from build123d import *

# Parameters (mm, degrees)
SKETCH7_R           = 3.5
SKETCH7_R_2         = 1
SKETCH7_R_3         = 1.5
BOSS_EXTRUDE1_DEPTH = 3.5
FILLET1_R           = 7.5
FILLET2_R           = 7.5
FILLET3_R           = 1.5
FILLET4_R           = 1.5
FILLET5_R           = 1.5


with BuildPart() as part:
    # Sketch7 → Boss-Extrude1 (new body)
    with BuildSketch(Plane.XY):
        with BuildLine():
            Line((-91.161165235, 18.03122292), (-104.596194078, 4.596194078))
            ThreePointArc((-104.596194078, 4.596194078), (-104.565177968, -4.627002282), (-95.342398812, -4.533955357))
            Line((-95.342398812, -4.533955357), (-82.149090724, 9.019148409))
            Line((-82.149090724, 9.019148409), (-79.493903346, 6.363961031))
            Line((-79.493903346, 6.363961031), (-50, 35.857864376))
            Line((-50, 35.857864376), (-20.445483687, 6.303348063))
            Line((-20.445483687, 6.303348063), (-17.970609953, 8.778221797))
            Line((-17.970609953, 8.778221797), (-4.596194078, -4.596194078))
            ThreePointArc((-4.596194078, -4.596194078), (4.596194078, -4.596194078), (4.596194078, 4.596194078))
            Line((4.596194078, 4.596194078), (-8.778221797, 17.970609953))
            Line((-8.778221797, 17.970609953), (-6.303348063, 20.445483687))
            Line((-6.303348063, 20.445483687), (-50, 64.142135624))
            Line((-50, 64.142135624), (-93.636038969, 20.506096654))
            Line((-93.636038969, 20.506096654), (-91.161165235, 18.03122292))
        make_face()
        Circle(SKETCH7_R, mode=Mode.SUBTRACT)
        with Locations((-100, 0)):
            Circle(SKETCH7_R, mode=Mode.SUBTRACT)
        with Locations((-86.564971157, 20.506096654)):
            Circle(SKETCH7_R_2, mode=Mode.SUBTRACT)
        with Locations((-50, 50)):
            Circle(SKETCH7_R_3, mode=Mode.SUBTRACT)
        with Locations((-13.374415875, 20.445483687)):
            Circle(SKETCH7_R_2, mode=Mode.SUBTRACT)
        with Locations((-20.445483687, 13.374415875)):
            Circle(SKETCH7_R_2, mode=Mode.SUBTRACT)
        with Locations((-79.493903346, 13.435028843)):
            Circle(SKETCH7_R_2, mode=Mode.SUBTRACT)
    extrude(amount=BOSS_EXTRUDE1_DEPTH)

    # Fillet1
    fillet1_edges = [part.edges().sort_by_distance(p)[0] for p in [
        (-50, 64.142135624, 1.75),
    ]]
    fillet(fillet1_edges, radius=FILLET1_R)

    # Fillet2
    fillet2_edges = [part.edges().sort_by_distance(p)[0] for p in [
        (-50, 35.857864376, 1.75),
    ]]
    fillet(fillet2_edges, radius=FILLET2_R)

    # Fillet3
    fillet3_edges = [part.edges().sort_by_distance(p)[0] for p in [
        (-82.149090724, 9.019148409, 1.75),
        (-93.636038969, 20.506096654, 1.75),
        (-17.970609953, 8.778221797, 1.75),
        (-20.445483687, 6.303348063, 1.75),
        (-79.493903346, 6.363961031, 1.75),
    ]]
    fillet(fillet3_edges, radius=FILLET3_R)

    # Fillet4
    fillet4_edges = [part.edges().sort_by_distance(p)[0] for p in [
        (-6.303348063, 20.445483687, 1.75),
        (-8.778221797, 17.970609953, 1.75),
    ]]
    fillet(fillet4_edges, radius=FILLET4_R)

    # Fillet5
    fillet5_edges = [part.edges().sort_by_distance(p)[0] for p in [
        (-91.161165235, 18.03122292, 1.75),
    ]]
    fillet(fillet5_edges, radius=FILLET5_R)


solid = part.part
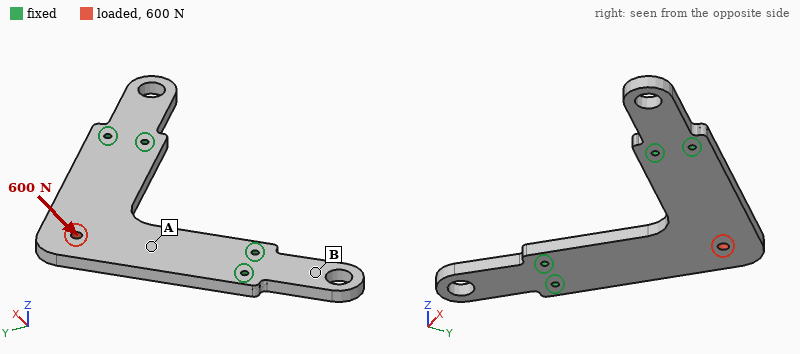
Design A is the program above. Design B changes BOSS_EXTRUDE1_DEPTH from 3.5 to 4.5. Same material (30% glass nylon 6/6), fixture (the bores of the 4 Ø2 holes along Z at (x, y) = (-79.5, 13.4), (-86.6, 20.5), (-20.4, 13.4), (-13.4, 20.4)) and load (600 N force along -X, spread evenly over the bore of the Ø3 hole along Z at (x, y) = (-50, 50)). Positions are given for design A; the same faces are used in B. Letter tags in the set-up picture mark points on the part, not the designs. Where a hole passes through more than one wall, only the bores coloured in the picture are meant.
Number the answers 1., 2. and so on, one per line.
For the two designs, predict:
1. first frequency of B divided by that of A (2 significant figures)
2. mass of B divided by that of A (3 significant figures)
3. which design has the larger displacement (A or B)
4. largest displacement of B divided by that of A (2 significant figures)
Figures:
1. 1.3
2. 1.29
3. A
4. 0.78
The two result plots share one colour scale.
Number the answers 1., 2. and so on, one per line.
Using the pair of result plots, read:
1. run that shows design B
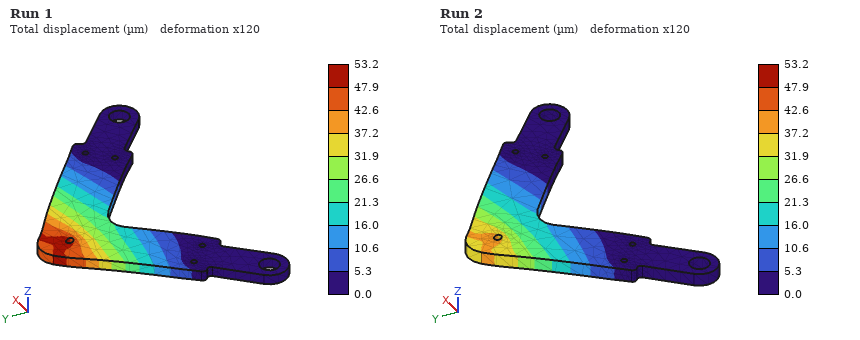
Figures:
1. Run 2
